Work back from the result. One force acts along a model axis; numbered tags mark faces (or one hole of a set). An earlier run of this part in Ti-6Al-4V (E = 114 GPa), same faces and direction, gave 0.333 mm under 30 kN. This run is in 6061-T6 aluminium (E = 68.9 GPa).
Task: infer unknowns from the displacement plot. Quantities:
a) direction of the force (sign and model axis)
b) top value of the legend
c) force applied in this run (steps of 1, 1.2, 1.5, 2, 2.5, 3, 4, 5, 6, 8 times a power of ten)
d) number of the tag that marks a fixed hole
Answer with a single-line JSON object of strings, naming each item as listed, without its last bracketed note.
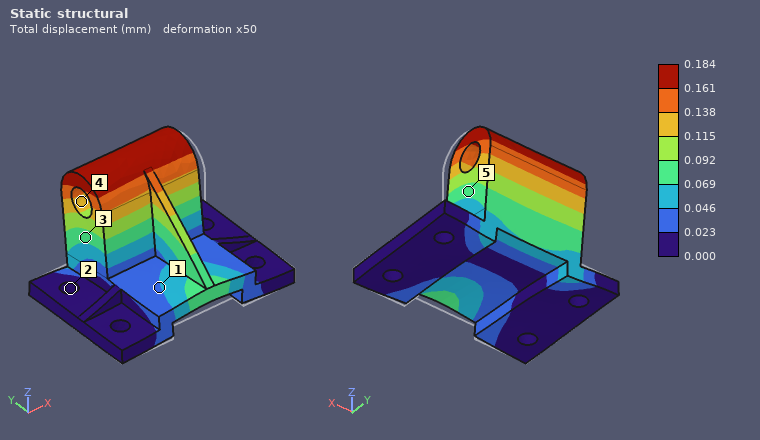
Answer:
{"direction of the force": "+Y", "top value of the legend": "0.184 mm", "force applied in this run": "10 kN", "number of the tag that marks a fixed hole": "2"}
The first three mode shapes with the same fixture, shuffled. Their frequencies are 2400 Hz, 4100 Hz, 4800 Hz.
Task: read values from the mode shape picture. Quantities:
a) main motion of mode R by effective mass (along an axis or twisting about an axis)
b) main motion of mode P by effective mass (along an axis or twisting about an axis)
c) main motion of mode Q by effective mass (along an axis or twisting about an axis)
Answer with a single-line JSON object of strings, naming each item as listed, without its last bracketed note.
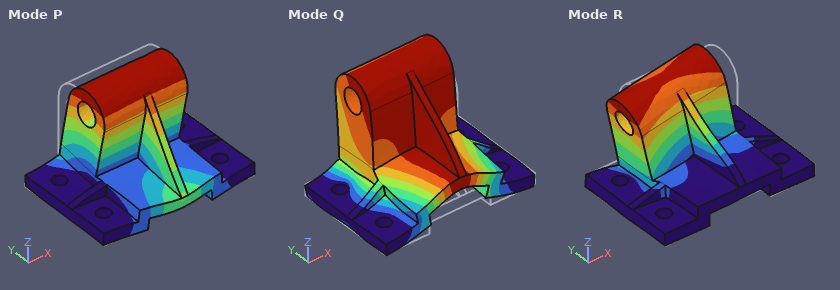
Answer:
{"main motion of mode R by effective mass": "along X", "main motion of mode P by effective mass": "along Y", "main motion of mode Q by effective mass": "along Z"}
